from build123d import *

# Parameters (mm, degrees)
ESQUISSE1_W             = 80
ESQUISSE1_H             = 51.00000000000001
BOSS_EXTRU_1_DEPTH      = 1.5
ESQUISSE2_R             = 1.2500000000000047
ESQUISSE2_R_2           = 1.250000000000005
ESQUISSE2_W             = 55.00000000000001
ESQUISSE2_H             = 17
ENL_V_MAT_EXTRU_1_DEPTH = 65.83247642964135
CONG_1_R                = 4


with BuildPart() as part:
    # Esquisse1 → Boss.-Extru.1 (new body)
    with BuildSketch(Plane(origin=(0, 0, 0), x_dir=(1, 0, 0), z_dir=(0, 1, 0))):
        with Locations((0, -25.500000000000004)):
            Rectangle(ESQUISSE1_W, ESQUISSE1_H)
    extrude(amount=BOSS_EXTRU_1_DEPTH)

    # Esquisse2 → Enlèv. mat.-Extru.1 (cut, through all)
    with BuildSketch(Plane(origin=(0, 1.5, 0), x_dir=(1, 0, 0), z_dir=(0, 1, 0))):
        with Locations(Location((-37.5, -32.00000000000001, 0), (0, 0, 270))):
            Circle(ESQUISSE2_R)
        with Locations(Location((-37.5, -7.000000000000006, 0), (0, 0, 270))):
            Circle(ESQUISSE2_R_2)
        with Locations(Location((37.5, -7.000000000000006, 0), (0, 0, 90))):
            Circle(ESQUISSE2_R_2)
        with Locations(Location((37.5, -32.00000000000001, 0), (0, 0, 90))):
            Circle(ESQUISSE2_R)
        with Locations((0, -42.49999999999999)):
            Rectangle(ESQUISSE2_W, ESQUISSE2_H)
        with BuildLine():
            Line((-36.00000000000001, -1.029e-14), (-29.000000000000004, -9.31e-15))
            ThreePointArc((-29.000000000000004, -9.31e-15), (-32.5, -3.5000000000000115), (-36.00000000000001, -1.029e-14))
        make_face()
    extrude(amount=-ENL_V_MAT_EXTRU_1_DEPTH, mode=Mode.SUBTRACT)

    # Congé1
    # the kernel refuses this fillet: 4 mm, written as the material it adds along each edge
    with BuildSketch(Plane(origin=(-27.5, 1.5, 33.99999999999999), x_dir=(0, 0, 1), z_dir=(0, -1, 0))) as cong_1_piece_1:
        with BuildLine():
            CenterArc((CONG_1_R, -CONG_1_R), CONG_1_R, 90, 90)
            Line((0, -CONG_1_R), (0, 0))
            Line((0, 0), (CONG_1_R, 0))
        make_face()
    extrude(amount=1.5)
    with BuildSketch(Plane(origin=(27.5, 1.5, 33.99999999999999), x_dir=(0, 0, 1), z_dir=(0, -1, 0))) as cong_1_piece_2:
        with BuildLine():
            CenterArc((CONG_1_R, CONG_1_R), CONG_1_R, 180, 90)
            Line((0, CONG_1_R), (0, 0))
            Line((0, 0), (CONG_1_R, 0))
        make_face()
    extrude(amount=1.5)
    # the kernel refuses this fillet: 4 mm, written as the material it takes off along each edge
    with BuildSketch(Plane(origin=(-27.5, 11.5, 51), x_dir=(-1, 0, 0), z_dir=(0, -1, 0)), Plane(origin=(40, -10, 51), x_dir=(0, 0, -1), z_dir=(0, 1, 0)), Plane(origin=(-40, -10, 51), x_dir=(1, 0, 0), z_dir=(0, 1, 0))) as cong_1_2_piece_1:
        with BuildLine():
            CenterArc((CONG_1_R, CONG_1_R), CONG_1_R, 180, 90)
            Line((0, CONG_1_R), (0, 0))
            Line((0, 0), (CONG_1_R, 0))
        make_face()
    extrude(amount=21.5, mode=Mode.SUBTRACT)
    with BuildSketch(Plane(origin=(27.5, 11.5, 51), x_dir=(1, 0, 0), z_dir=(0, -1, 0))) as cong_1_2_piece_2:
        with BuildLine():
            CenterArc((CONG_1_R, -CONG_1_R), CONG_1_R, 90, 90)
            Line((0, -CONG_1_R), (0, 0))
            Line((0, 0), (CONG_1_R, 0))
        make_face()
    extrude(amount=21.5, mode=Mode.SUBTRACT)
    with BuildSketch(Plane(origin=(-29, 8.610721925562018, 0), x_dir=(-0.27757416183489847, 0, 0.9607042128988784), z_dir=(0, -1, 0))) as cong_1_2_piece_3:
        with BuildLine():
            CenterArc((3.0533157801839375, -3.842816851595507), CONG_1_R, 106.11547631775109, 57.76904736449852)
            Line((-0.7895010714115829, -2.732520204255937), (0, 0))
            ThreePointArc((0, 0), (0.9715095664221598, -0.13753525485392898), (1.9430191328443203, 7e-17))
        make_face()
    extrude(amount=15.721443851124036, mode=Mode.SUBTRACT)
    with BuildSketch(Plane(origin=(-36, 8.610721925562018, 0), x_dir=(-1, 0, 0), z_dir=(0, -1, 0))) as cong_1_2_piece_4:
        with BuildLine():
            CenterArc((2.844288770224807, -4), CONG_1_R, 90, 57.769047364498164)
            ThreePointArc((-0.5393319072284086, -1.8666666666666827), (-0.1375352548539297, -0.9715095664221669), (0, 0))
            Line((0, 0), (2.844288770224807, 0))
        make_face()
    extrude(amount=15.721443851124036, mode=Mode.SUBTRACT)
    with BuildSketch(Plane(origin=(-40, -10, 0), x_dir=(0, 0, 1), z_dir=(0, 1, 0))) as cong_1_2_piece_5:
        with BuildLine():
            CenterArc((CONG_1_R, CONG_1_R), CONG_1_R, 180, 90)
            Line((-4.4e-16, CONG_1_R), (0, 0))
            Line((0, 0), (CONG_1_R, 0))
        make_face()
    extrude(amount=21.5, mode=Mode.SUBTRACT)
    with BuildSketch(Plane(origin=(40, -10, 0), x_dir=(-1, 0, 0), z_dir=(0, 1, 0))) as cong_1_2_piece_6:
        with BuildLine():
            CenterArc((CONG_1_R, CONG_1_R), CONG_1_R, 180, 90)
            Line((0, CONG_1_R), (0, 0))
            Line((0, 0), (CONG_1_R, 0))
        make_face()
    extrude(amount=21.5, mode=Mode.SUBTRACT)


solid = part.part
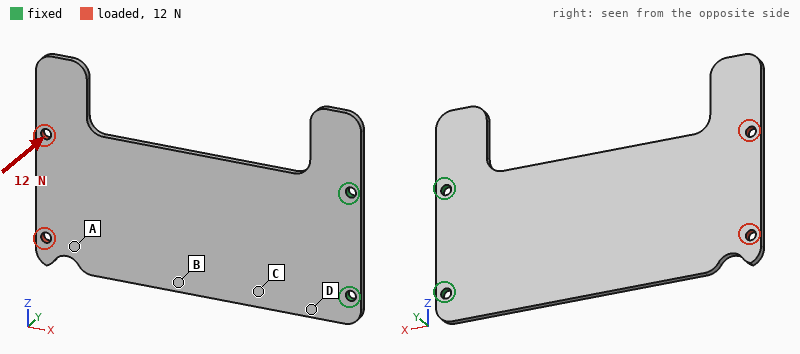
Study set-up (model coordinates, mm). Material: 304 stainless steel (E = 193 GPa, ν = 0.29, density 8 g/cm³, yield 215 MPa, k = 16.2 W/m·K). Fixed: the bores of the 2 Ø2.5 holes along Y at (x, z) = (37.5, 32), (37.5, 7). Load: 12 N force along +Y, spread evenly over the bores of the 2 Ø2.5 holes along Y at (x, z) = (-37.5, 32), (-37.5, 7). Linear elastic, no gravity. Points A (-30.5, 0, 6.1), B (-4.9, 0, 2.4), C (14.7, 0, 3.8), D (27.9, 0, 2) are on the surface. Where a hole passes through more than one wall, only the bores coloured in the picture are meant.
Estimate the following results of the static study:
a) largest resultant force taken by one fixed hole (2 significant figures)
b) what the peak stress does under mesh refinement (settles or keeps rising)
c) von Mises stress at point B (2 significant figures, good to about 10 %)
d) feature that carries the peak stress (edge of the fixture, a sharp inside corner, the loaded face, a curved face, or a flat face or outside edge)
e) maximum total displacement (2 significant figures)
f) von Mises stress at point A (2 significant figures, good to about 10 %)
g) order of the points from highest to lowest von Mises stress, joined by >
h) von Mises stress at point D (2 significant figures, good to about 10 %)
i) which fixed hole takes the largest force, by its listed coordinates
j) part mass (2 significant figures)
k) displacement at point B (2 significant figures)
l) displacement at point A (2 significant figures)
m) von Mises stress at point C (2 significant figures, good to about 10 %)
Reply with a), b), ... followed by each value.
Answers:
a) 6.6 N
b) keeps rising
c) 31 MPa
d) edge of the fixture
e) 0.97 mm
f) 10 MPa
g) D > C > B > A
h) 62 MPa
i) (37.5, 7)
j) 37 g
k) 0.36 mm
l) 0.79 mm
m) 48 MPa
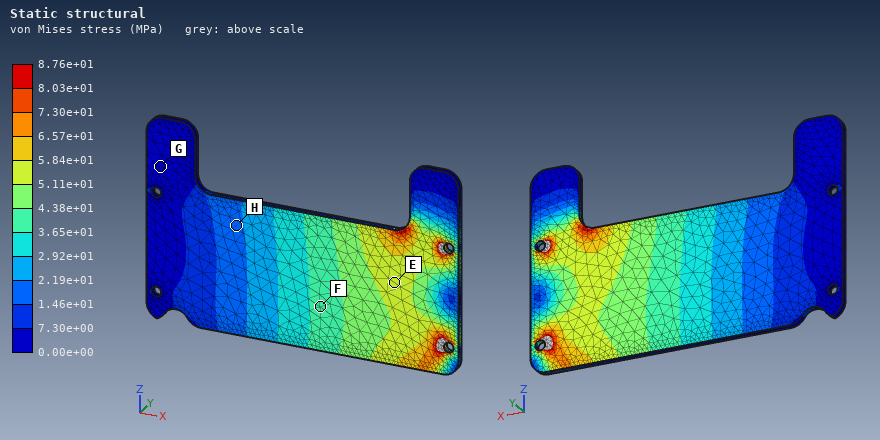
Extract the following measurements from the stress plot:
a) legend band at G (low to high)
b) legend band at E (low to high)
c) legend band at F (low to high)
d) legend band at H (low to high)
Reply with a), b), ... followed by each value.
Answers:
a) 0.00e+00 to 7.30e+00 MPa
b) 5.11e+01 to 5.84e+01 MPa
c) 3.65e+01 to 4.38e+01 MPa
d) 1.46e+01 to 2.19e+01 MPa
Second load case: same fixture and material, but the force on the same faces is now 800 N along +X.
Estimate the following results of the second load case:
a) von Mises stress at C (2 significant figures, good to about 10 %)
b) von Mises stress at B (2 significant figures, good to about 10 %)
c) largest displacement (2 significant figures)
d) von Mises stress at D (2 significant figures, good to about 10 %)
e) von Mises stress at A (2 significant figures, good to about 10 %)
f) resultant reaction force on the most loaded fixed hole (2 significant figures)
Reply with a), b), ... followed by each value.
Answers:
a) 11 MPa
b) 9.8 MPa
c) 14 µm
d) 12 MPa
e) 25 MPa
f) 410 N
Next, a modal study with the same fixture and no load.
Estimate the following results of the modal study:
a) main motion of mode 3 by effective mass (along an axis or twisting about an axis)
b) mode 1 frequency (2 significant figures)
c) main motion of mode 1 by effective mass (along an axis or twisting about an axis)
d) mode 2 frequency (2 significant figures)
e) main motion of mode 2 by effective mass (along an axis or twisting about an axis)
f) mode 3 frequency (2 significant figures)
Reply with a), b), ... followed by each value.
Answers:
a) along Y
b) 180 Hz
c) along Y
d) 690 Hz
e) twisting about X
f) 1200 Hz
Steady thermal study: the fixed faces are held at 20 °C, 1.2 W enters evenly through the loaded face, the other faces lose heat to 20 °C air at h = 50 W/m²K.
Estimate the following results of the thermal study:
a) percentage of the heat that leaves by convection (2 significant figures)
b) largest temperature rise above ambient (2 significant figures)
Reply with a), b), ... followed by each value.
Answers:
a) 99 %
b) 26 K
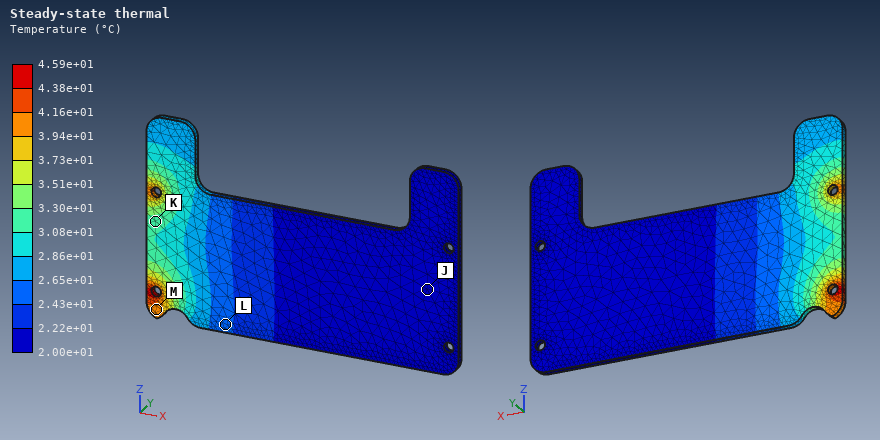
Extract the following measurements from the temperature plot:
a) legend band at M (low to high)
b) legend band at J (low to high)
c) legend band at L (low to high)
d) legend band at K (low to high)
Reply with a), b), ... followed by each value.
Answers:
a) 3.94e+01 to 4.16e+01 °C
b) 2.00e+01 to 2.22e+01 °C
c) 2.43e+01 to 2.65e+01 °C
d) 3.08e+01 to 3.30e+01 °C
